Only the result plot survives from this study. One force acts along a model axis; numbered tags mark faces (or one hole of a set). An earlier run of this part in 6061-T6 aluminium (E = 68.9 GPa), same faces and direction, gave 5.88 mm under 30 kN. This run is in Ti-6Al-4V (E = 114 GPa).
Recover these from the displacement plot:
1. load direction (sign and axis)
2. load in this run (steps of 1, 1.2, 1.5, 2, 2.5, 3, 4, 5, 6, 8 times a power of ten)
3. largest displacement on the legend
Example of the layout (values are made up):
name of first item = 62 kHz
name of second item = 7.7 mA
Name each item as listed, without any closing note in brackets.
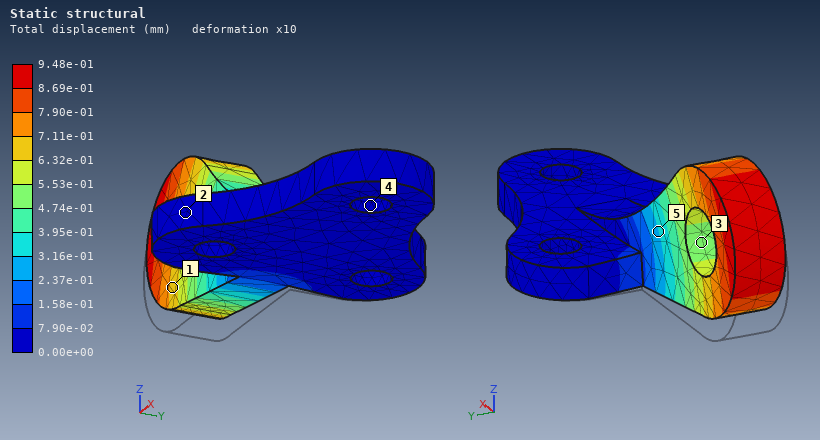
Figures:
load direction = +Z
load in this run = 8 kN
largest displacement on the legend = 9.48e-01 mm
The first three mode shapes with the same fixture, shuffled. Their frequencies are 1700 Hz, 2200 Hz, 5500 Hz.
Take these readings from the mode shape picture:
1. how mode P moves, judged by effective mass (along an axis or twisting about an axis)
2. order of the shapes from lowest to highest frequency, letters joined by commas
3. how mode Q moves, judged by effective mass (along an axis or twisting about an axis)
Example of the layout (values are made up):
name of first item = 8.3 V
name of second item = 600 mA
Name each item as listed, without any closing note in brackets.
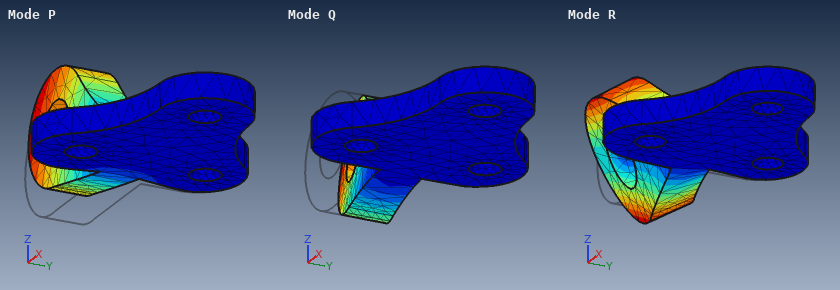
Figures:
how mode P moves, judged by effective mass = along Z
order of the shapes from lowest to highest frequency, letters joined by commas = P, Q, R
how mode Q moves, judged by effective mass = along Y
